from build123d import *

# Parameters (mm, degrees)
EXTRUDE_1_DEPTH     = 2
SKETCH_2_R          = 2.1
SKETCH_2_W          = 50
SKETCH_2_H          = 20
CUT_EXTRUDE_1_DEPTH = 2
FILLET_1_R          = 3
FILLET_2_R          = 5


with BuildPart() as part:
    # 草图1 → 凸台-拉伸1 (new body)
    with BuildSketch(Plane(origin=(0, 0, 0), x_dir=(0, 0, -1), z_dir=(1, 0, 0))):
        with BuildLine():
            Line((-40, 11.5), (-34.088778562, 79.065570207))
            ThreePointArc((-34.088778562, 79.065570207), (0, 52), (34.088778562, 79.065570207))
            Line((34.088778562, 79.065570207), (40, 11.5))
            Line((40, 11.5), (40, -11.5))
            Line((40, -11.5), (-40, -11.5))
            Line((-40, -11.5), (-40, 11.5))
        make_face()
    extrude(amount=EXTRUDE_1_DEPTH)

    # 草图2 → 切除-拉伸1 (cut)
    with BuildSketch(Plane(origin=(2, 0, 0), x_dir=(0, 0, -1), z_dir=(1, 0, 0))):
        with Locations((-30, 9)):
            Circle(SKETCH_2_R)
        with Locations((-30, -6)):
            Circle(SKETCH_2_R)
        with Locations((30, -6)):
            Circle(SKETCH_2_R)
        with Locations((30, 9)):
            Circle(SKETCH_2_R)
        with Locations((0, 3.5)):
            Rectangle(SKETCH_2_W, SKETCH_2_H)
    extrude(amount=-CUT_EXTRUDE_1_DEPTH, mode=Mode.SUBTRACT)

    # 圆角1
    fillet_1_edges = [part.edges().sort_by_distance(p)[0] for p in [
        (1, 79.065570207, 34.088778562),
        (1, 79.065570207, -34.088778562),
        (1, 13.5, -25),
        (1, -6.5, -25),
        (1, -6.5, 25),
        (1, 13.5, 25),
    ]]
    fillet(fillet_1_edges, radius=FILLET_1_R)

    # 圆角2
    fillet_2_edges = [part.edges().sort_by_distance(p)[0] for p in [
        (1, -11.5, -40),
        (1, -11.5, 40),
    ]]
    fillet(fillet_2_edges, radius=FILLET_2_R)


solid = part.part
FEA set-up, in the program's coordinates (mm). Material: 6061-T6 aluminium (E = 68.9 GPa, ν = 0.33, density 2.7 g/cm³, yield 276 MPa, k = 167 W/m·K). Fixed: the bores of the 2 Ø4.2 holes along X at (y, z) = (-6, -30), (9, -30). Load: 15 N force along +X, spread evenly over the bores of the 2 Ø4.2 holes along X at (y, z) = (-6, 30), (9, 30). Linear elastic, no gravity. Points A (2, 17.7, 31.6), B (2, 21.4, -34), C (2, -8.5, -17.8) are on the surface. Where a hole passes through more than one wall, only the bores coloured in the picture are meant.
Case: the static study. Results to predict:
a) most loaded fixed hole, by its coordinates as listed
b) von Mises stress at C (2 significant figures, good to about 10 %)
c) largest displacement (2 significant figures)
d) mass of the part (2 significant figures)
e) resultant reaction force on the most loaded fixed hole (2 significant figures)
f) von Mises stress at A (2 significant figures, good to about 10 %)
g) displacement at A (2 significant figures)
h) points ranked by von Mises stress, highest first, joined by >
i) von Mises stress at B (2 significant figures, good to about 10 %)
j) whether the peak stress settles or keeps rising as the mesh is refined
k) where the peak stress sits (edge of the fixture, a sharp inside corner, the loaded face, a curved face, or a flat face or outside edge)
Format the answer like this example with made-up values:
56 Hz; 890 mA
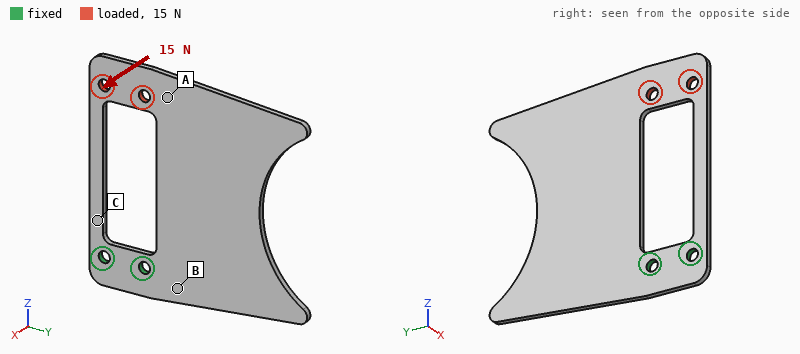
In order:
(-6, -30); 57 MPa; 1.2 mm; 24 g; 11 N; 9.8 MPa; 0.90 mm; C > B > A; 29 MPa; keeps rising; edge of the fixture
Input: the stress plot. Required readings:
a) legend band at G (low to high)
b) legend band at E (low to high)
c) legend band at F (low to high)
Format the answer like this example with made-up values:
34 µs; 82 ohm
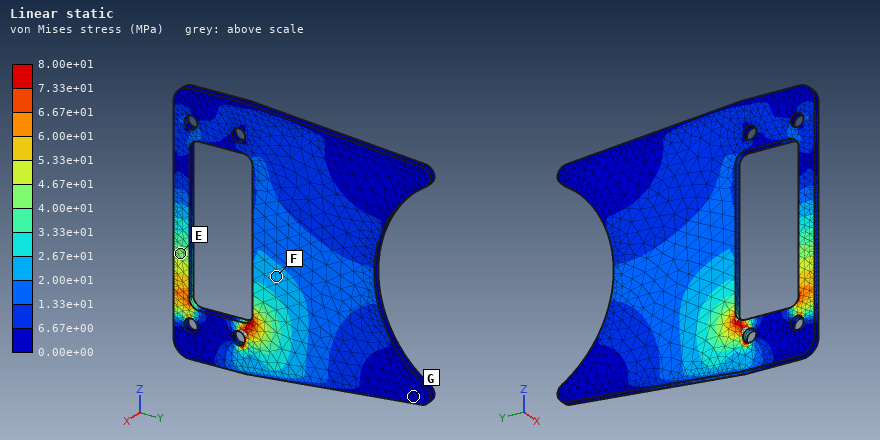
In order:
0.00e+00 to 6.67e+00 MPa; 4.00e+01 to 4.67e+01 MPa; 2.00e+01 to 2.67e+01 MPa
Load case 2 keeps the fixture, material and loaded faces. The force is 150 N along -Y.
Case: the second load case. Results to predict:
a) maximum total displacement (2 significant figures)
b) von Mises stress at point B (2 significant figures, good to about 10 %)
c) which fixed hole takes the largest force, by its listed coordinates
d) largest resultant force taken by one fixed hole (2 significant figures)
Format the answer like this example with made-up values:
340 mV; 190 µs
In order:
0.22 mm; 22 MPa; (9, -30); 490 N
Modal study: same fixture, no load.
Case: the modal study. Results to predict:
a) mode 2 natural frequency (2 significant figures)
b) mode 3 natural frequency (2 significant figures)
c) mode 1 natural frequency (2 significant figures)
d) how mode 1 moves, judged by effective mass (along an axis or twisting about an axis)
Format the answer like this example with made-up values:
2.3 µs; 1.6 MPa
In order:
420 Hz; 930 Hz; 200 Hz; along X
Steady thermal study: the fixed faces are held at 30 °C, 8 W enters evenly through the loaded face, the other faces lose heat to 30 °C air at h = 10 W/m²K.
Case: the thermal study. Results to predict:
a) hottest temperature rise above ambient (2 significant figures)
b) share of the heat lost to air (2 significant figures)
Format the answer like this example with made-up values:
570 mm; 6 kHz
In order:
56 K; 27 %
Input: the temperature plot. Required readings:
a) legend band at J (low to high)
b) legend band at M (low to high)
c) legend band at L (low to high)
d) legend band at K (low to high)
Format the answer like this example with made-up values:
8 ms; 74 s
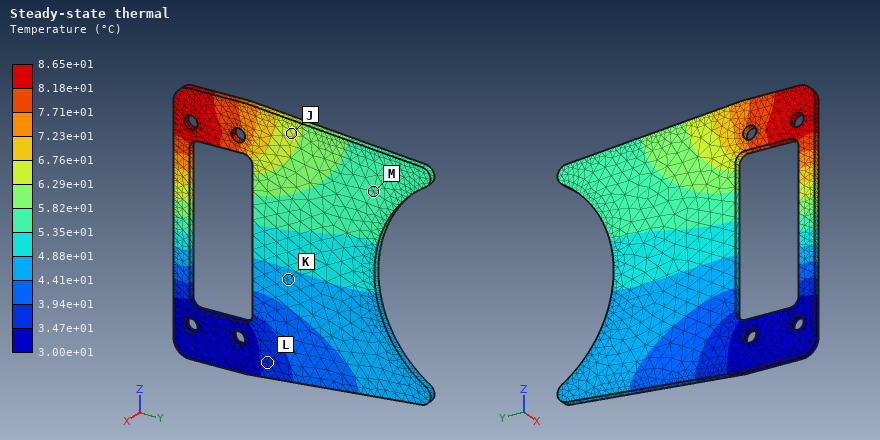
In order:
6.29e+01 to 6.76e+01 °C; 5.35e+01 to 5.82e+01 °C; 3.47e+01 to 3.94e+01 °C; 4.41e+01 to 4.88e+01 °C
